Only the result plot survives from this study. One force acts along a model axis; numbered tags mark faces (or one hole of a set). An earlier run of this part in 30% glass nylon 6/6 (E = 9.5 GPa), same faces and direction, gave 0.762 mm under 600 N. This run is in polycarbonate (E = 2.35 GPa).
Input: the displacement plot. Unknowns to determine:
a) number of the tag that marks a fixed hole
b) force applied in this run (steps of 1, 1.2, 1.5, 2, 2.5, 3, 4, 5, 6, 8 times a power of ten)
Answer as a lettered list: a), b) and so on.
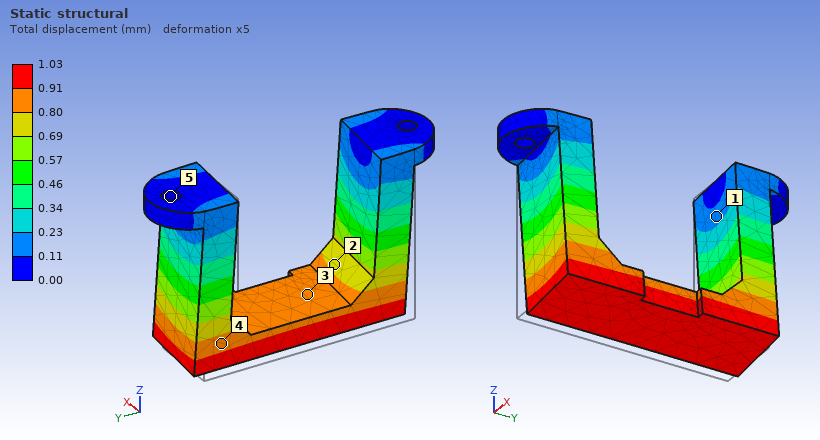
a) 5
b) 200 N
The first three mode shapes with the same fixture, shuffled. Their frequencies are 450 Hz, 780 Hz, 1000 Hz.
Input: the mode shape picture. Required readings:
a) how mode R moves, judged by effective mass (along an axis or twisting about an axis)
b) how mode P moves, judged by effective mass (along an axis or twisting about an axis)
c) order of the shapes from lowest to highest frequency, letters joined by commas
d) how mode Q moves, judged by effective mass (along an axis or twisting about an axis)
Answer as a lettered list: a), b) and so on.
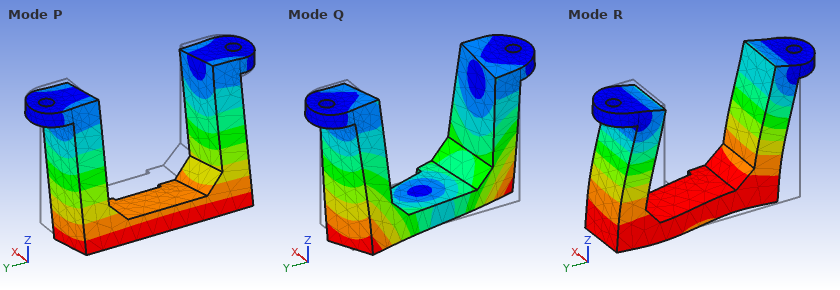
a) along Y
b) along X
c) P, R, Q
d) twisting about Z
